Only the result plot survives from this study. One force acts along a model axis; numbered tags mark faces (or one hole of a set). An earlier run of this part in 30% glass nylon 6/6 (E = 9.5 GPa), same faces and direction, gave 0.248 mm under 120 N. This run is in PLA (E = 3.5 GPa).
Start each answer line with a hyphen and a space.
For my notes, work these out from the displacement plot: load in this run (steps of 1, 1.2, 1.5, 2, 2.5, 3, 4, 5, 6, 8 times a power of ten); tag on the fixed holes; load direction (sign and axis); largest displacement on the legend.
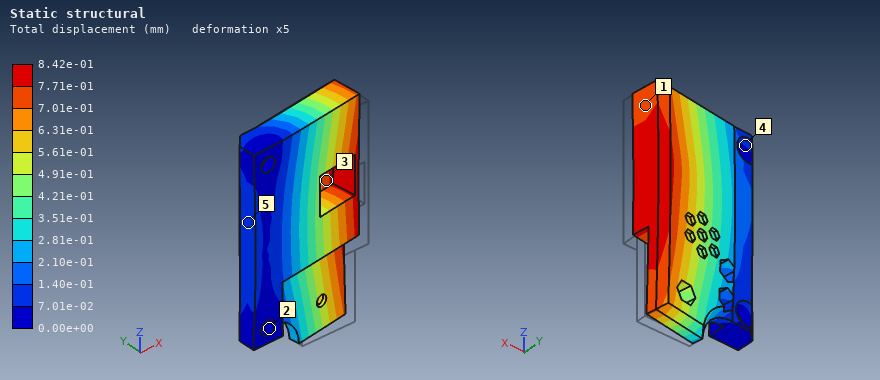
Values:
- 150 N
- 2
- +Y
- 8.42e-01 mm
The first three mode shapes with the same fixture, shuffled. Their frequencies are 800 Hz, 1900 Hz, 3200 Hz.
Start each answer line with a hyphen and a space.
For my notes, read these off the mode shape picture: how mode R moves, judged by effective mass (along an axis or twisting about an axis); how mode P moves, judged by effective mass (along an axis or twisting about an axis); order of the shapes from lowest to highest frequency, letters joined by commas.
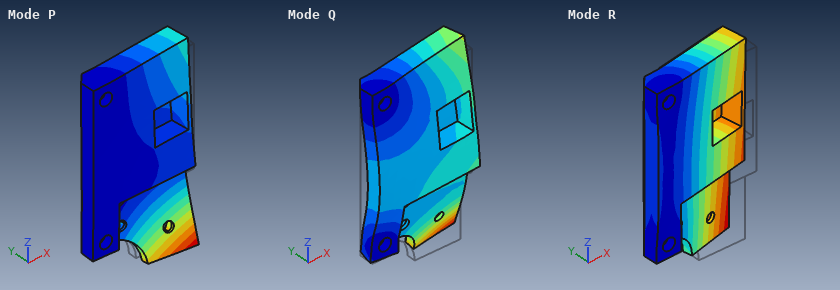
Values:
- along Y
- twisting about X
- R, P, Q
